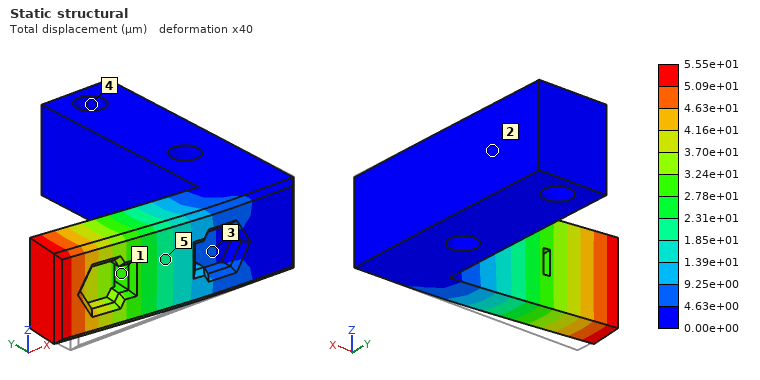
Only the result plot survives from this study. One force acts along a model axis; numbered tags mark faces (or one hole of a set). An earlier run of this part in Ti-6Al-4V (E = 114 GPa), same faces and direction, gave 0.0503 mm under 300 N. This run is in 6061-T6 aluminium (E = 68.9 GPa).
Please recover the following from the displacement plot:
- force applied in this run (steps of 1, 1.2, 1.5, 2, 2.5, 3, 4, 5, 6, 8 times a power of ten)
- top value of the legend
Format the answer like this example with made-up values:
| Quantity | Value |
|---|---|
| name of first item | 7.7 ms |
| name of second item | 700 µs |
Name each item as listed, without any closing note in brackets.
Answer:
| Quantity | Value |
|---|---|
| force applied in this run | 200 N |
| top value of the legend | 5.55e+01 µm |
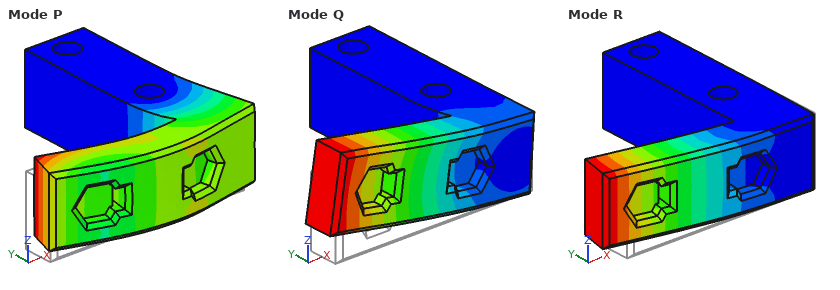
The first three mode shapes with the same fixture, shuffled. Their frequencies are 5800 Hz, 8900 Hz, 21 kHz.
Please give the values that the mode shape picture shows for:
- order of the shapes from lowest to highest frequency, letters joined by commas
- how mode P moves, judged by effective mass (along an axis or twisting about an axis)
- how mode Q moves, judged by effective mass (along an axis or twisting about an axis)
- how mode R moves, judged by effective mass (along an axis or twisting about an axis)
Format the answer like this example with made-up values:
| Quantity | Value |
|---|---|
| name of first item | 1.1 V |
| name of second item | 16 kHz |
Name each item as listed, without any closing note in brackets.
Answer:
| Quantity | Value |
|---|---|
| order of the shapes from lowest to highest frequency, letters joined by commas | R, Q, P |
| how mode P moves, judged by effective mass | along X |
| how mode Q moves, judged by effective mass | along Z |
| how mode R moves, judged by effective mass | along Y |
